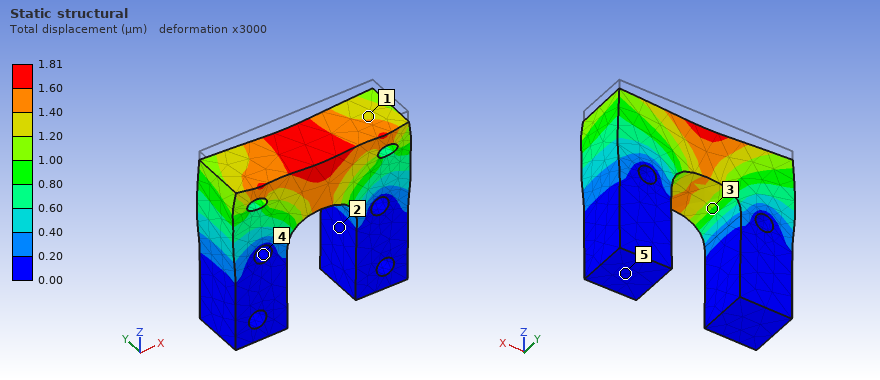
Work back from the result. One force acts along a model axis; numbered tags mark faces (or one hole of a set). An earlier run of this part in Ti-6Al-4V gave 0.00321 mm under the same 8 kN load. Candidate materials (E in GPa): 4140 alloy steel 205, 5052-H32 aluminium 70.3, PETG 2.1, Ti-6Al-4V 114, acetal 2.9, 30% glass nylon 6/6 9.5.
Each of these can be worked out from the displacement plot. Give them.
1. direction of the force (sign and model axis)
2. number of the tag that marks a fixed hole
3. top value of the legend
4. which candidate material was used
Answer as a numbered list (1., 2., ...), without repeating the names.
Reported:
1. -Z
2. 4
3. 1.81 µm
4. 4140 alloy steel
